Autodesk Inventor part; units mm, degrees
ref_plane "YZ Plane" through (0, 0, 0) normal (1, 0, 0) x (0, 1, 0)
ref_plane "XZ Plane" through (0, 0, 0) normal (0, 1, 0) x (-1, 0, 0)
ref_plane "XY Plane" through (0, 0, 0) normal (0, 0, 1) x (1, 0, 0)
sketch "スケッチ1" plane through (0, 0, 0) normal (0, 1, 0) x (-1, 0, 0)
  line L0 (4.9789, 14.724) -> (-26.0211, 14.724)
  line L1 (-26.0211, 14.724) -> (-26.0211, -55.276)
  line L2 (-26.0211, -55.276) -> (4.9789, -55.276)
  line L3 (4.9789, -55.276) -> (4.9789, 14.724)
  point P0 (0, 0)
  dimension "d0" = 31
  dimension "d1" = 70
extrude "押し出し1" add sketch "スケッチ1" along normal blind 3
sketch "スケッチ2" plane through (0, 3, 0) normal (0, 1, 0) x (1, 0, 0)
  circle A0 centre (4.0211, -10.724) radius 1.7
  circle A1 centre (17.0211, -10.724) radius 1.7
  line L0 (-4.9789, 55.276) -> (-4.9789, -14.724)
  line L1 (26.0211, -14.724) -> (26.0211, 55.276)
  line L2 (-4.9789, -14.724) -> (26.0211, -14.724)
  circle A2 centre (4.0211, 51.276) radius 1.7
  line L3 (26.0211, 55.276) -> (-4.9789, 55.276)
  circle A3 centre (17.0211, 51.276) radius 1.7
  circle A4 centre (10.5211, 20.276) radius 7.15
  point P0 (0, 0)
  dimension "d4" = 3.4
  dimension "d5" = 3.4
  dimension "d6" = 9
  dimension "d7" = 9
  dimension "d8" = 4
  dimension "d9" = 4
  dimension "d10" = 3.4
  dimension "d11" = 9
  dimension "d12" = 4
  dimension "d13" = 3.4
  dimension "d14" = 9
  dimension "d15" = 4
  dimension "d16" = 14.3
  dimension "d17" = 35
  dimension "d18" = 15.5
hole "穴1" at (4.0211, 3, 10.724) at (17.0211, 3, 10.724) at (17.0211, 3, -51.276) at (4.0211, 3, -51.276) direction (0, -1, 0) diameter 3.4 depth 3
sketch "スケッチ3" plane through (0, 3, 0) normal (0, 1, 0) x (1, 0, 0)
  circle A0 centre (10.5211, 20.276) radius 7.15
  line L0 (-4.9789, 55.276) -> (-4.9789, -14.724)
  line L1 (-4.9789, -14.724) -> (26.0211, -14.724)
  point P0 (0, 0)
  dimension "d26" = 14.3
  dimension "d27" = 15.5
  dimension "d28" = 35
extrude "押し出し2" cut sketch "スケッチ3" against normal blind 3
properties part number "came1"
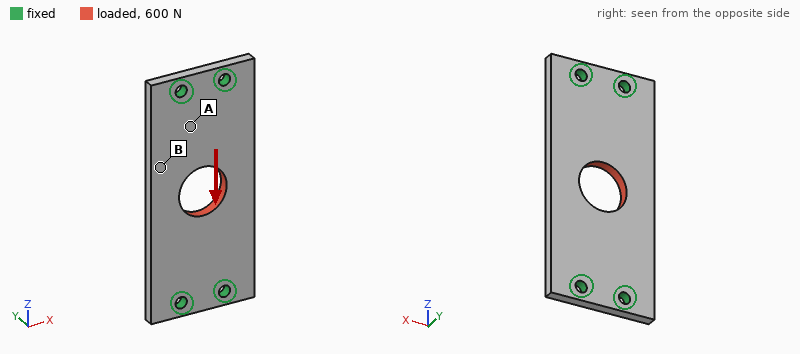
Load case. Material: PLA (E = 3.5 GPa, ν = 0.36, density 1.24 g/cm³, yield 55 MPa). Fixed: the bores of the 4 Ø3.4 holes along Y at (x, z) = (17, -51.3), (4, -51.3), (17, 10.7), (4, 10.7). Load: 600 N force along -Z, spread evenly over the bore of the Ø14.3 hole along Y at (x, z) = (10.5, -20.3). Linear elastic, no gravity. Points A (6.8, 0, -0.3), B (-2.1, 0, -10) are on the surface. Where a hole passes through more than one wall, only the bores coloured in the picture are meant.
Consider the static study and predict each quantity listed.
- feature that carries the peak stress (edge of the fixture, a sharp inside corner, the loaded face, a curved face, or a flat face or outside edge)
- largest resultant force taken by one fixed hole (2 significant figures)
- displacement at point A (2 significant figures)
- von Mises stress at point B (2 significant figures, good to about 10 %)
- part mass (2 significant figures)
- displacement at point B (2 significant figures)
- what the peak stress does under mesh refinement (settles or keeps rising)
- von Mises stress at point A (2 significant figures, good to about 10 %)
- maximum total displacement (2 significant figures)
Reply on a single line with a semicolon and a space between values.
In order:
edge of the fixture; 150 N; 14 µm; 2.0 MPa; 7.3 g; 22 µm; keeps rising; 4.3 MPa; 36 µm
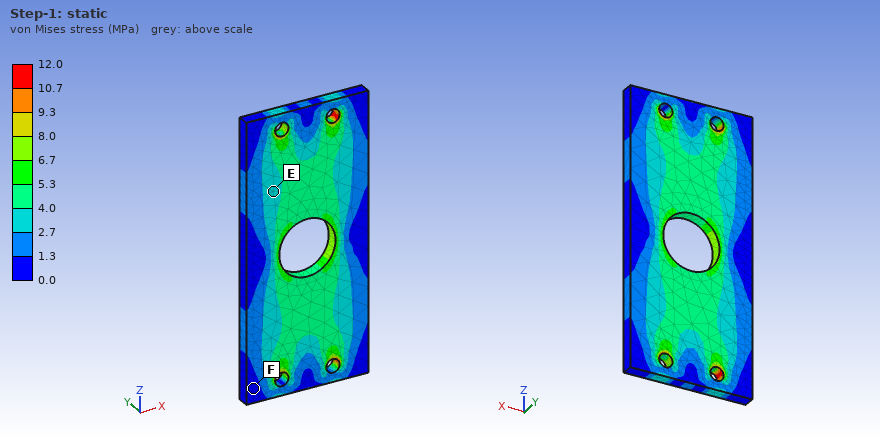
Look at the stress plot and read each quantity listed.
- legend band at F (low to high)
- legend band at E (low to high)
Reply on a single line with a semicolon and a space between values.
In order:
0.0 to 1.3 MPa; 2.7 to 4.0 MPa
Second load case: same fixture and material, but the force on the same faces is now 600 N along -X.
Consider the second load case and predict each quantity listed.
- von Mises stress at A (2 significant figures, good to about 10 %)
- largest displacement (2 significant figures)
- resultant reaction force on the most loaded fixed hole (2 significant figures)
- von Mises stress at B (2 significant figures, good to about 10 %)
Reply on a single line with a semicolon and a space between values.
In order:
8.7 MPa; 0.14 mm; 240 N; 6.1 MPa
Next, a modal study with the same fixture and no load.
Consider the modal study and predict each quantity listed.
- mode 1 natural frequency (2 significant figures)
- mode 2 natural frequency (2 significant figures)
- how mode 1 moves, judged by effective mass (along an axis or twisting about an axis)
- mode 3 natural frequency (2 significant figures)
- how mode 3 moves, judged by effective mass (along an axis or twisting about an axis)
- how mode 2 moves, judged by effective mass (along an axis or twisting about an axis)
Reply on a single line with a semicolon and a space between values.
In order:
1400 Hz; 2000 Hz; along Y; 3500 Hz; twisting about X; twisting about Z
